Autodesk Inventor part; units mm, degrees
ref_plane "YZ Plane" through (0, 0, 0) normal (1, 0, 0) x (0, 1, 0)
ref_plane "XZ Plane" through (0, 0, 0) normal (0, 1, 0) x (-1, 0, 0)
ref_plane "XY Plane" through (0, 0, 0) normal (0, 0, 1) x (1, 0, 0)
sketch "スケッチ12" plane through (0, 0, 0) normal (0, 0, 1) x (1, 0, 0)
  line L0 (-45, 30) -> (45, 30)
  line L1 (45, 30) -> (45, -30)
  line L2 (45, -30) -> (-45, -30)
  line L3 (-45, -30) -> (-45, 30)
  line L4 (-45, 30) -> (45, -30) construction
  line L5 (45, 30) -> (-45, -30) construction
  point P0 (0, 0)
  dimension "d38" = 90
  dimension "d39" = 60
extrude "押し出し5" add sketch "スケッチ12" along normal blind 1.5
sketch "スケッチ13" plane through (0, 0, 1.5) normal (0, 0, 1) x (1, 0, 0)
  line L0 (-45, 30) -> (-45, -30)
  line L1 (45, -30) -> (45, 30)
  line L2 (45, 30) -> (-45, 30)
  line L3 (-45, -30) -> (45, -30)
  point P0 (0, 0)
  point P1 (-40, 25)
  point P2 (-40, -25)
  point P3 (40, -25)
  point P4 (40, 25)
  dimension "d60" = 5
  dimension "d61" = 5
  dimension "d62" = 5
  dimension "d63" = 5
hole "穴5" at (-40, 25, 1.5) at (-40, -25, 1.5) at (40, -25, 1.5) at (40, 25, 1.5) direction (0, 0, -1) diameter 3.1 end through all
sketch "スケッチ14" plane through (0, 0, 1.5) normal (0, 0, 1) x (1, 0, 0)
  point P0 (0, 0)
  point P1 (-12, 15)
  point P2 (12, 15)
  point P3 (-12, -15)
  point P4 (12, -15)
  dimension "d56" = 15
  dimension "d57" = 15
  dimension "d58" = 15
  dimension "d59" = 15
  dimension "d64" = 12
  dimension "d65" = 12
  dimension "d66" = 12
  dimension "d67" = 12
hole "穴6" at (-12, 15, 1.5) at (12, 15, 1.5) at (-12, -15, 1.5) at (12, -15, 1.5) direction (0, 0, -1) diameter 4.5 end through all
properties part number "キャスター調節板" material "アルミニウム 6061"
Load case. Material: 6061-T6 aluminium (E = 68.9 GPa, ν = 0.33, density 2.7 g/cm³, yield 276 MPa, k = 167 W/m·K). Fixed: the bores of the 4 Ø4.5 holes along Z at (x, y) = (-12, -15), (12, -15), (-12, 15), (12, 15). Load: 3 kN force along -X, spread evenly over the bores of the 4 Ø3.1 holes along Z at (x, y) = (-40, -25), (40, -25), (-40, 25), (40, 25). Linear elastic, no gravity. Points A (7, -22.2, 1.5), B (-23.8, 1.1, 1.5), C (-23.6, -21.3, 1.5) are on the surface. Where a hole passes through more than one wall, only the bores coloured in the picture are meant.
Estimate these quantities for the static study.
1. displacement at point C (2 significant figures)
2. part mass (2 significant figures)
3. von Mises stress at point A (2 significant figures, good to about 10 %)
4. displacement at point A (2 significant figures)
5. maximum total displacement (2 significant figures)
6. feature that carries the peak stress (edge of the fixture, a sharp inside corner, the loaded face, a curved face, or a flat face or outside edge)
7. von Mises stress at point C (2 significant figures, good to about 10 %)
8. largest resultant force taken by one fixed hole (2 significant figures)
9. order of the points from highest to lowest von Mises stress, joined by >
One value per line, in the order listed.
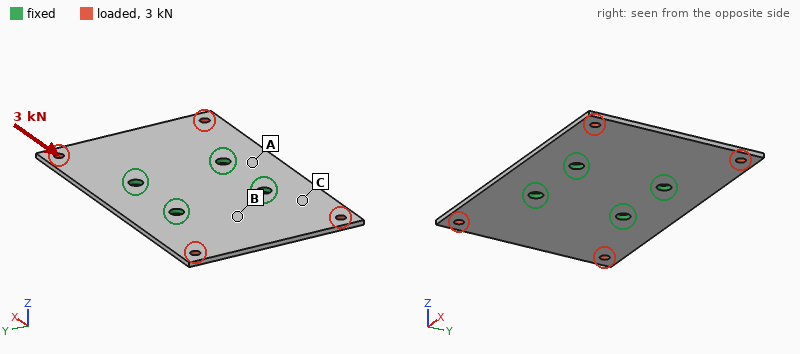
6.5 µm
21 g
16 MPa
3.2 µm
21 µm
the loaded face
30 MPa
750 N
C > A > B
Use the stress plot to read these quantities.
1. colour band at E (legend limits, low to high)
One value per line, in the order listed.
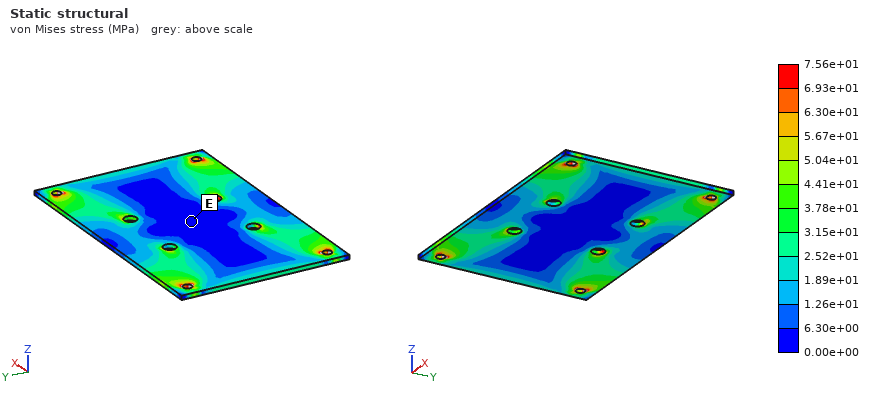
0.00e+00 to 6.30e+00 MPa
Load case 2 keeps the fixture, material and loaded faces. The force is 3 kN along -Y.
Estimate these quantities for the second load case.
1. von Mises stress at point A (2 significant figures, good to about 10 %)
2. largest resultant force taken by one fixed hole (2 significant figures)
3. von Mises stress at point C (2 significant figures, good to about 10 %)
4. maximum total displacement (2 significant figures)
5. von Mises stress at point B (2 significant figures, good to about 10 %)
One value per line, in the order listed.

23 MPa
880 N
24 MPa
46 µm
46 MPa
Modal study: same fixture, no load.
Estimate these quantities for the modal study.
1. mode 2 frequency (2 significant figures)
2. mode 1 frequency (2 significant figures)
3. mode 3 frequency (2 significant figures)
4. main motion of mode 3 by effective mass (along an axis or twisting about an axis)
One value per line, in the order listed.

1200 Hz
1200 Hz
1800 Hz
twisting about X
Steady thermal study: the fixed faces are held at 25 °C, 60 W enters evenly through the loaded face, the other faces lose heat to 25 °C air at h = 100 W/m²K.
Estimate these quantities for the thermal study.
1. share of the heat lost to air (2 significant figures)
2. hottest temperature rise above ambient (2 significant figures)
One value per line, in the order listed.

39 %
74 K
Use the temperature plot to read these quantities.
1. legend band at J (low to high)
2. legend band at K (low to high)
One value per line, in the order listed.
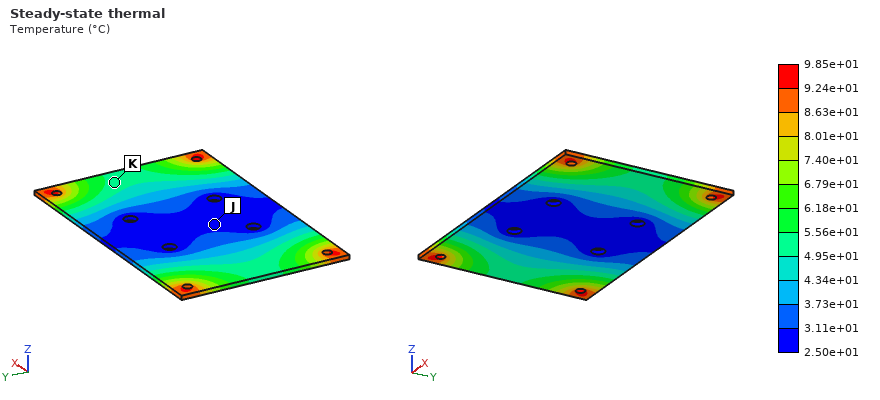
2.50e+01 to 3.11e+01 °C
4.95e+01 to 5.56e+01 °C
